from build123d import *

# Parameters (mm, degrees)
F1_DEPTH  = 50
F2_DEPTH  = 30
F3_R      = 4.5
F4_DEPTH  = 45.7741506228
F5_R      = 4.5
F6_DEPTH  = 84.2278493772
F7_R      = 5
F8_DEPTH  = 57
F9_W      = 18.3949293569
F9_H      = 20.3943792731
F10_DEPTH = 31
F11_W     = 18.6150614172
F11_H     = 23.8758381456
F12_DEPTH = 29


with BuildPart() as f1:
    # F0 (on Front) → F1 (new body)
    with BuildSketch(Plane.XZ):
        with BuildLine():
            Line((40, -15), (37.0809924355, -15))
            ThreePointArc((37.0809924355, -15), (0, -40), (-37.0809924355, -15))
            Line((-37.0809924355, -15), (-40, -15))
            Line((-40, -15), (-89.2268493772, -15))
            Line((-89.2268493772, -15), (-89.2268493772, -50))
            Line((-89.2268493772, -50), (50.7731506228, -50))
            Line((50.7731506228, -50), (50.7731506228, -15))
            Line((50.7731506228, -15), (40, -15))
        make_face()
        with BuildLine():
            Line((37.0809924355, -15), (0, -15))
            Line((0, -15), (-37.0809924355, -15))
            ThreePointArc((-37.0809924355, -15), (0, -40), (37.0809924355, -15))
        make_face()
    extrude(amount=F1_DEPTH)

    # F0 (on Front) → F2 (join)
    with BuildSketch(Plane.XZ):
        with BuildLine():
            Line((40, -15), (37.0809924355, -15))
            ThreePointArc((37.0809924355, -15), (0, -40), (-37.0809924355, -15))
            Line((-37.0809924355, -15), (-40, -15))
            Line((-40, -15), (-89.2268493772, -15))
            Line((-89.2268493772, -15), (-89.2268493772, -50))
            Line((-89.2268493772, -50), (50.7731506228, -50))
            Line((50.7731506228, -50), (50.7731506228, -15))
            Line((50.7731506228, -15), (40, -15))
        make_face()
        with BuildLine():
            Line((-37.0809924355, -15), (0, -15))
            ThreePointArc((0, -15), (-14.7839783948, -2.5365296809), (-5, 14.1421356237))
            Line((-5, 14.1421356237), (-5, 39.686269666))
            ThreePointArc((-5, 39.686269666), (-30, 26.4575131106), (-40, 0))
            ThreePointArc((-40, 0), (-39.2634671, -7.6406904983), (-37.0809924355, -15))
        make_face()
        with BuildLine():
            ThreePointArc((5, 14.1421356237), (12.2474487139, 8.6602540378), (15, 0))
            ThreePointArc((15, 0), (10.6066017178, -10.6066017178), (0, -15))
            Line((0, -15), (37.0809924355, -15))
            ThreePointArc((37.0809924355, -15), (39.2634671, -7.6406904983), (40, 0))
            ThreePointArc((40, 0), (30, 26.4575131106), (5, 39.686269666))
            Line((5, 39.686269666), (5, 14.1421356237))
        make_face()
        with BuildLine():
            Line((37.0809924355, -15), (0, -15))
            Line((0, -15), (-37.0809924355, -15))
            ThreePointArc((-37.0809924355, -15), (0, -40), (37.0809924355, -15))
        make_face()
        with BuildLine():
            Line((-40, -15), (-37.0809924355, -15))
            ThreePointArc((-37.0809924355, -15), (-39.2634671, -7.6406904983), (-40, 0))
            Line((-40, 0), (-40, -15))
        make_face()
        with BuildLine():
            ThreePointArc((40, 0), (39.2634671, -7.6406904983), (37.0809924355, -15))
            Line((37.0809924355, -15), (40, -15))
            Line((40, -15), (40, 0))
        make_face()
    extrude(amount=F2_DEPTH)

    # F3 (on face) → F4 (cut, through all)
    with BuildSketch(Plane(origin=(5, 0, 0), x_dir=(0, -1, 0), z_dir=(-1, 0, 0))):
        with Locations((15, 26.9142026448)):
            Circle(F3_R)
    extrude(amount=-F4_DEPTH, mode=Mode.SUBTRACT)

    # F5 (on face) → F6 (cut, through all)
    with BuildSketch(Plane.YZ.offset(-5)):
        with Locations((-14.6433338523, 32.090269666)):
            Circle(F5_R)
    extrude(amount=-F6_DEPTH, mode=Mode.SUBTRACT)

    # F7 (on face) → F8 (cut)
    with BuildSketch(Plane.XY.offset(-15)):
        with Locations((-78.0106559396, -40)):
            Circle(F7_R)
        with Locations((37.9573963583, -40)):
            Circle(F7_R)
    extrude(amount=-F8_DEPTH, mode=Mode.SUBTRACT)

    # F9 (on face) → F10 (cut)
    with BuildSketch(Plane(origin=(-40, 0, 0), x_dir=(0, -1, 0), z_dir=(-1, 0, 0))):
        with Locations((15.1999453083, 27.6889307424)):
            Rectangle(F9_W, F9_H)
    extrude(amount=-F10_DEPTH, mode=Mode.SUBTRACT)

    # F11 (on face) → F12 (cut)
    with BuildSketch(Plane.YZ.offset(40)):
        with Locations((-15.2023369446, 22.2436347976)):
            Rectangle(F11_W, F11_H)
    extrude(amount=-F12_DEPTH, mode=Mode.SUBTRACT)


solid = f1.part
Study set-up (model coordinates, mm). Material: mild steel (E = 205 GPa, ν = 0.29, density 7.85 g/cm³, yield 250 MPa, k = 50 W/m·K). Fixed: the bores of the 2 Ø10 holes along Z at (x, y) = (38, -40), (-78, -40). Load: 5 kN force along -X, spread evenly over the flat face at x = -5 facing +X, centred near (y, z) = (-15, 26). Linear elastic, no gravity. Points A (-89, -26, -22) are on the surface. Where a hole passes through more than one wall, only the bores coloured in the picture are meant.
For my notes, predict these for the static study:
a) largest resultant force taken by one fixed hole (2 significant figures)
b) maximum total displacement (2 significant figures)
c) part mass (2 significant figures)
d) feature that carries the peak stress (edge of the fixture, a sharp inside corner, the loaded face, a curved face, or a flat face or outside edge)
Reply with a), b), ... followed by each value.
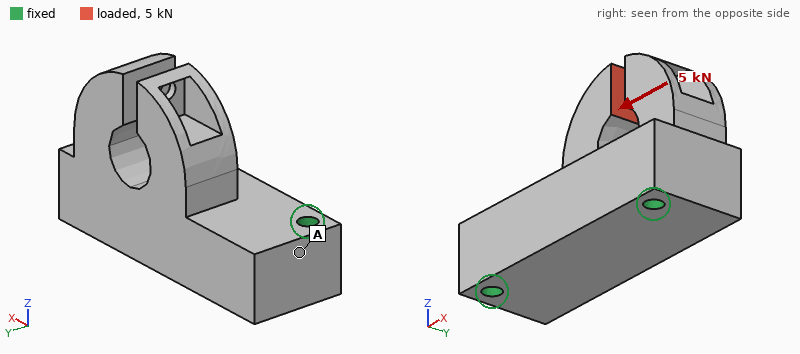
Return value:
a) 4.0 kN
b) 51 µm
c) 2.4 kg
d) a curved face
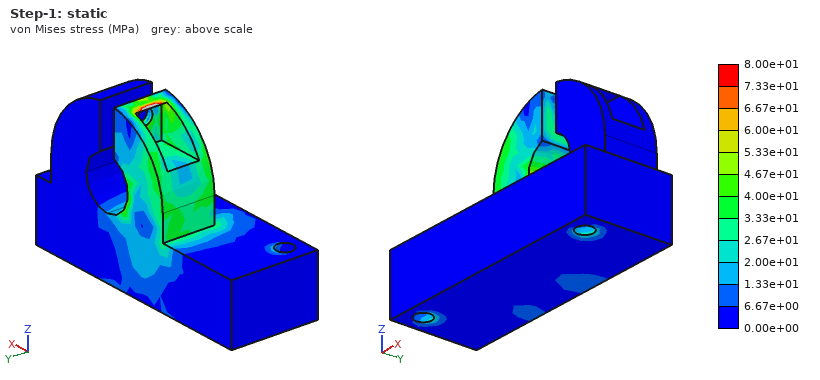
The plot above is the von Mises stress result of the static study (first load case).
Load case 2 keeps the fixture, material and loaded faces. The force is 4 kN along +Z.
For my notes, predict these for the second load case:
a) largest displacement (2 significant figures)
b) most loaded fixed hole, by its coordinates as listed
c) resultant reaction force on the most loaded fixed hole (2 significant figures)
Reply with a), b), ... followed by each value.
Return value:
a) 29 µm
b) (38, -40)
c) 2.6 kN
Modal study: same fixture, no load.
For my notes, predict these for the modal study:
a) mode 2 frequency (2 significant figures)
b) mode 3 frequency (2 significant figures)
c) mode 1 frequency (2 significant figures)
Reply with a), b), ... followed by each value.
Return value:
a) 5500 Hz
b) 5700 Hz
c) 4000 Hz
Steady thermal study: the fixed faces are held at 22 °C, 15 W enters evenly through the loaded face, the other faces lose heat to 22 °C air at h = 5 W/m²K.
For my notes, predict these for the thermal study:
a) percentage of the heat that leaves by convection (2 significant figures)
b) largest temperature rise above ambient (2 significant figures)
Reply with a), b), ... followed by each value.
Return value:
a) 7.0 %
b) 39 K
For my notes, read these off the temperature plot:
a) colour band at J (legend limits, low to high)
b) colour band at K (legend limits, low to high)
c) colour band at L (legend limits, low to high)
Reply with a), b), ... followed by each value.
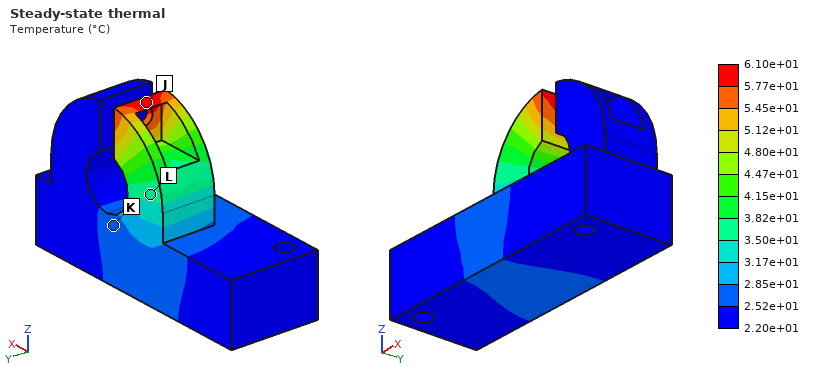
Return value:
a) 5.77e+01 to 6.10e+01 °C
b) 2.52e+01 to 2.85e+01 °C
c) 3.50e+01 to 3.82e+01 °C
